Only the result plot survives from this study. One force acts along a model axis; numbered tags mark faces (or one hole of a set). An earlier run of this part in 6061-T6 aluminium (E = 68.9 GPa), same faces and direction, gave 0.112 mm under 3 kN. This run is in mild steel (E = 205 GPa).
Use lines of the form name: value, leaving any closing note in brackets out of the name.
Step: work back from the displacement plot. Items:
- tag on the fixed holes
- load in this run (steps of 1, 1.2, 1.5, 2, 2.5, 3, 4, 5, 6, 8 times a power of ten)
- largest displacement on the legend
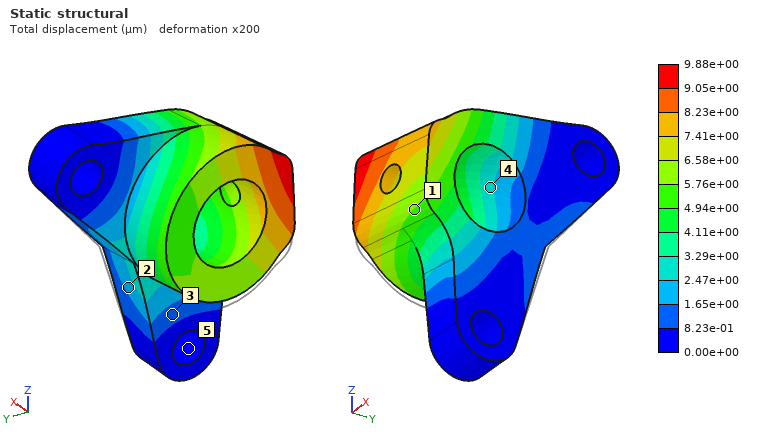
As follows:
tag on the fixed holes: 5
load in this run: 800 N
largest displacement on the legend: 9.88e+00 µm
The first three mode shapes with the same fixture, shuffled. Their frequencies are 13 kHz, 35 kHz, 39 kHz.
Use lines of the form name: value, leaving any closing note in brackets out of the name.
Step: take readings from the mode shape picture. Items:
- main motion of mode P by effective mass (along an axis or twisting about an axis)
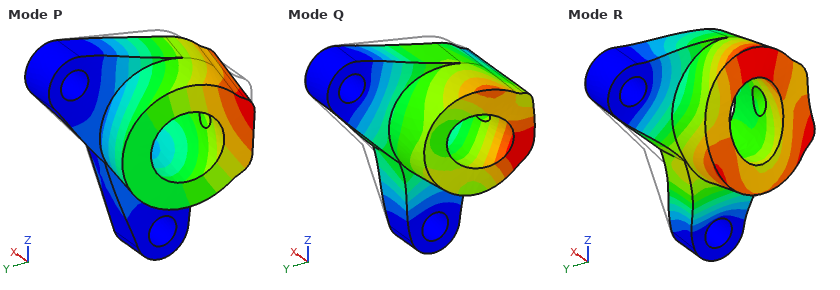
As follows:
main motion of mode P by effective mass: along X
